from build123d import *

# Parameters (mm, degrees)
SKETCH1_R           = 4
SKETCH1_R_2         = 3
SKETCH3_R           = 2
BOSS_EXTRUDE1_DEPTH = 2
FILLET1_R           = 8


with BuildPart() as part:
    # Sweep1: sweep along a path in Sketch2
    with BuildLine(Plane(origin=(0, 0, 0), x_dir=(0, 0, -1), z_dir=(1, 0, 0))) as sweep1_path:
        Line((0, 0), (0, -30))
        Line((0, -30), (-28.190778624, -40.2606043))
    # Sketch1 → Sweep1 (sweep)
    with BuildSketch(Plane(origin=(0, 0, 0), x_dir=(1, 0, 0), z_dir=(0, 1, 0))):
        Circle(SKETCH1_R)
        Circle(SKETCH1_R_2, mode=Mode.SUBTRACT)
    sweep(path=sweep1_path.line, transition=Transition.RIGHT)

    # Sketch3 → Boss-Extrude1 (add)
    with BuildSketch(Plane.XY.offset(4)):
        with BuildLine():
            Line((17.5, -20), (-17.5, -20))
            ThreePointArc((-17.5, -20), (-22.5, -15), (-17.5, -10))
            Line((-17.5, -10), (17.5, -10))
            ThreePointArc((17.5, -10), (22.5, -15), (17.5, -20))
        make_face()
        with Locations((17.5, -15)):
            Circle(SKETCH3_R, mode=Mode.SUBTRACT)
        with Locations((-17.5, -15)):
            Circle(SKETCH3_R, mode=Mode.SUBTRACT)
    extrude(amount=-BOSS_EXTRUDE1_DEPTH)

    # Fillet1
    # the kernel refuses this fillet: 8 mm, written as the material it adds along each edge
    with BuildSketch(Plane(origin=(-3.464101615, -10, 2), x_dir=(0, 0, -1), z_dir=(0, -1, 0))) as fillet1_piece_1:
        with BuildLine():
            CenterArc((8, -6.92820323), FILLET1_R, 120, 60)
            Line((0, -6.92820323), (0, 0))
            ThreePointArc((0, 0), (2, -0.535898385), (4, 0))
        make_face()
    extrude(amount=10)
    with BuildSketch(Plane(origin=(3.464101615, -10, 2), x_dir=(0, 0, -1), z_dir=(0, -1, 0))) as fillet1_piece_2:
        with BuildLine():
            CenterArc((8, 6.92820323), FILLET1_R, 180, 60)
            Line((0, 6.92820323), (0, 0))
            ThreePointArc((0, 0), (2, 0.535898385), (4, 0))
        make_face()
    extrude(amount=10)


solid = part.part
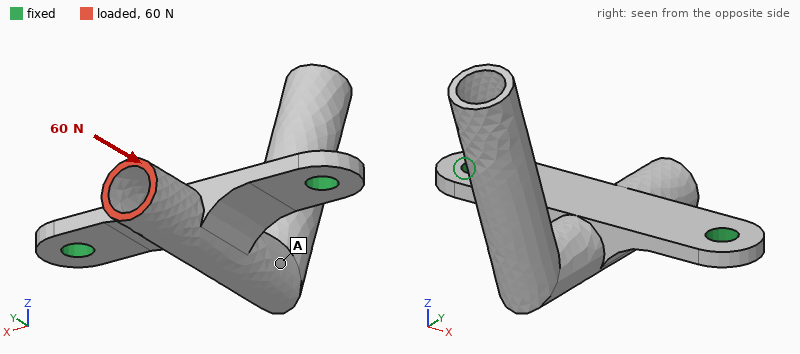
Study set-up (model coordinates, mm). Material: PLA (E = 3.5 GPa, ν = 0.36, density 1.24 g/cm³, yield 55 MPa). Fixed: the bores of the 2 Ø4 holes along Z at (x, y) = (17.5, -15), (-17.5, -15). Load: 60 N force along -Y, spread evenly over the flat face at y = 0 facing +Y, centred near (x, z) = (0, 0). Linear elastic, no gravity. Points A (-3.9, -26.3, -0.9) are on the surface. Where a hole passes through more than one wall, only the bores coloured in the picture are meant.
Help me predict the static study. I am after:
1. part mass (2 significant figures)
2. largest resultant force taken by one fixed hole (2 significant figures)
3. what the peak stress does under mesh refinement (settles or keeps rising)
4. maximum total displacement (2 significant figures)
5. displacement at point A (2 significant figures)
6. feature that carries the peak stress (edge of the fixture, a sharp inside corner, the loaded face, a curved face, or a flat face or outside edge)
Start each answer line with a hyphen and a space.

- 2.7 g
- 30 N
- keeps rising
- 0.76 mm
- 0.26 mm
- edge of the fixture
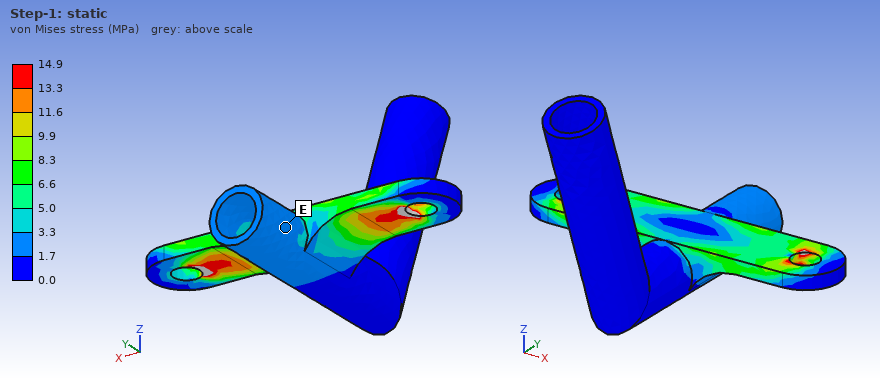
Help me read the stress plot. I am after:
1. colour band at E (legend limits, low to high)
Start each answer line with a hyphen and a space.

- 1.7 to 3.3 MPa
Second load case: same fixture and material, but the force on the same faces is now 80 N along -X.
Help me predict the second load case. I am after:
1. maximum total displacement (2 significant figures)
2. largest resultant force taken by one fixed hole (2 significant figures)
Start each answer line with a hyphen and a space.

- 0.26 mm
- 59 N
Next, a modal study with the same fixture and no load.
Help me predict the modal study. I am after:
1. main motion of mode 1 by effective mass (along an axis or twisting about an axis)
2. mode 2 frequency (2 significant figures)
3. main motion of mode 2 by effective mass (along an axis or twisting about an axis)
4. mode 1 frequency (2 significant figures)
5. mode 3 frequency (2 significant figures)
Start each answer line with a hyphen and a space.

- along Z
- 1100 Hz
- along X
- 560 Hz
- 2100 Hz
